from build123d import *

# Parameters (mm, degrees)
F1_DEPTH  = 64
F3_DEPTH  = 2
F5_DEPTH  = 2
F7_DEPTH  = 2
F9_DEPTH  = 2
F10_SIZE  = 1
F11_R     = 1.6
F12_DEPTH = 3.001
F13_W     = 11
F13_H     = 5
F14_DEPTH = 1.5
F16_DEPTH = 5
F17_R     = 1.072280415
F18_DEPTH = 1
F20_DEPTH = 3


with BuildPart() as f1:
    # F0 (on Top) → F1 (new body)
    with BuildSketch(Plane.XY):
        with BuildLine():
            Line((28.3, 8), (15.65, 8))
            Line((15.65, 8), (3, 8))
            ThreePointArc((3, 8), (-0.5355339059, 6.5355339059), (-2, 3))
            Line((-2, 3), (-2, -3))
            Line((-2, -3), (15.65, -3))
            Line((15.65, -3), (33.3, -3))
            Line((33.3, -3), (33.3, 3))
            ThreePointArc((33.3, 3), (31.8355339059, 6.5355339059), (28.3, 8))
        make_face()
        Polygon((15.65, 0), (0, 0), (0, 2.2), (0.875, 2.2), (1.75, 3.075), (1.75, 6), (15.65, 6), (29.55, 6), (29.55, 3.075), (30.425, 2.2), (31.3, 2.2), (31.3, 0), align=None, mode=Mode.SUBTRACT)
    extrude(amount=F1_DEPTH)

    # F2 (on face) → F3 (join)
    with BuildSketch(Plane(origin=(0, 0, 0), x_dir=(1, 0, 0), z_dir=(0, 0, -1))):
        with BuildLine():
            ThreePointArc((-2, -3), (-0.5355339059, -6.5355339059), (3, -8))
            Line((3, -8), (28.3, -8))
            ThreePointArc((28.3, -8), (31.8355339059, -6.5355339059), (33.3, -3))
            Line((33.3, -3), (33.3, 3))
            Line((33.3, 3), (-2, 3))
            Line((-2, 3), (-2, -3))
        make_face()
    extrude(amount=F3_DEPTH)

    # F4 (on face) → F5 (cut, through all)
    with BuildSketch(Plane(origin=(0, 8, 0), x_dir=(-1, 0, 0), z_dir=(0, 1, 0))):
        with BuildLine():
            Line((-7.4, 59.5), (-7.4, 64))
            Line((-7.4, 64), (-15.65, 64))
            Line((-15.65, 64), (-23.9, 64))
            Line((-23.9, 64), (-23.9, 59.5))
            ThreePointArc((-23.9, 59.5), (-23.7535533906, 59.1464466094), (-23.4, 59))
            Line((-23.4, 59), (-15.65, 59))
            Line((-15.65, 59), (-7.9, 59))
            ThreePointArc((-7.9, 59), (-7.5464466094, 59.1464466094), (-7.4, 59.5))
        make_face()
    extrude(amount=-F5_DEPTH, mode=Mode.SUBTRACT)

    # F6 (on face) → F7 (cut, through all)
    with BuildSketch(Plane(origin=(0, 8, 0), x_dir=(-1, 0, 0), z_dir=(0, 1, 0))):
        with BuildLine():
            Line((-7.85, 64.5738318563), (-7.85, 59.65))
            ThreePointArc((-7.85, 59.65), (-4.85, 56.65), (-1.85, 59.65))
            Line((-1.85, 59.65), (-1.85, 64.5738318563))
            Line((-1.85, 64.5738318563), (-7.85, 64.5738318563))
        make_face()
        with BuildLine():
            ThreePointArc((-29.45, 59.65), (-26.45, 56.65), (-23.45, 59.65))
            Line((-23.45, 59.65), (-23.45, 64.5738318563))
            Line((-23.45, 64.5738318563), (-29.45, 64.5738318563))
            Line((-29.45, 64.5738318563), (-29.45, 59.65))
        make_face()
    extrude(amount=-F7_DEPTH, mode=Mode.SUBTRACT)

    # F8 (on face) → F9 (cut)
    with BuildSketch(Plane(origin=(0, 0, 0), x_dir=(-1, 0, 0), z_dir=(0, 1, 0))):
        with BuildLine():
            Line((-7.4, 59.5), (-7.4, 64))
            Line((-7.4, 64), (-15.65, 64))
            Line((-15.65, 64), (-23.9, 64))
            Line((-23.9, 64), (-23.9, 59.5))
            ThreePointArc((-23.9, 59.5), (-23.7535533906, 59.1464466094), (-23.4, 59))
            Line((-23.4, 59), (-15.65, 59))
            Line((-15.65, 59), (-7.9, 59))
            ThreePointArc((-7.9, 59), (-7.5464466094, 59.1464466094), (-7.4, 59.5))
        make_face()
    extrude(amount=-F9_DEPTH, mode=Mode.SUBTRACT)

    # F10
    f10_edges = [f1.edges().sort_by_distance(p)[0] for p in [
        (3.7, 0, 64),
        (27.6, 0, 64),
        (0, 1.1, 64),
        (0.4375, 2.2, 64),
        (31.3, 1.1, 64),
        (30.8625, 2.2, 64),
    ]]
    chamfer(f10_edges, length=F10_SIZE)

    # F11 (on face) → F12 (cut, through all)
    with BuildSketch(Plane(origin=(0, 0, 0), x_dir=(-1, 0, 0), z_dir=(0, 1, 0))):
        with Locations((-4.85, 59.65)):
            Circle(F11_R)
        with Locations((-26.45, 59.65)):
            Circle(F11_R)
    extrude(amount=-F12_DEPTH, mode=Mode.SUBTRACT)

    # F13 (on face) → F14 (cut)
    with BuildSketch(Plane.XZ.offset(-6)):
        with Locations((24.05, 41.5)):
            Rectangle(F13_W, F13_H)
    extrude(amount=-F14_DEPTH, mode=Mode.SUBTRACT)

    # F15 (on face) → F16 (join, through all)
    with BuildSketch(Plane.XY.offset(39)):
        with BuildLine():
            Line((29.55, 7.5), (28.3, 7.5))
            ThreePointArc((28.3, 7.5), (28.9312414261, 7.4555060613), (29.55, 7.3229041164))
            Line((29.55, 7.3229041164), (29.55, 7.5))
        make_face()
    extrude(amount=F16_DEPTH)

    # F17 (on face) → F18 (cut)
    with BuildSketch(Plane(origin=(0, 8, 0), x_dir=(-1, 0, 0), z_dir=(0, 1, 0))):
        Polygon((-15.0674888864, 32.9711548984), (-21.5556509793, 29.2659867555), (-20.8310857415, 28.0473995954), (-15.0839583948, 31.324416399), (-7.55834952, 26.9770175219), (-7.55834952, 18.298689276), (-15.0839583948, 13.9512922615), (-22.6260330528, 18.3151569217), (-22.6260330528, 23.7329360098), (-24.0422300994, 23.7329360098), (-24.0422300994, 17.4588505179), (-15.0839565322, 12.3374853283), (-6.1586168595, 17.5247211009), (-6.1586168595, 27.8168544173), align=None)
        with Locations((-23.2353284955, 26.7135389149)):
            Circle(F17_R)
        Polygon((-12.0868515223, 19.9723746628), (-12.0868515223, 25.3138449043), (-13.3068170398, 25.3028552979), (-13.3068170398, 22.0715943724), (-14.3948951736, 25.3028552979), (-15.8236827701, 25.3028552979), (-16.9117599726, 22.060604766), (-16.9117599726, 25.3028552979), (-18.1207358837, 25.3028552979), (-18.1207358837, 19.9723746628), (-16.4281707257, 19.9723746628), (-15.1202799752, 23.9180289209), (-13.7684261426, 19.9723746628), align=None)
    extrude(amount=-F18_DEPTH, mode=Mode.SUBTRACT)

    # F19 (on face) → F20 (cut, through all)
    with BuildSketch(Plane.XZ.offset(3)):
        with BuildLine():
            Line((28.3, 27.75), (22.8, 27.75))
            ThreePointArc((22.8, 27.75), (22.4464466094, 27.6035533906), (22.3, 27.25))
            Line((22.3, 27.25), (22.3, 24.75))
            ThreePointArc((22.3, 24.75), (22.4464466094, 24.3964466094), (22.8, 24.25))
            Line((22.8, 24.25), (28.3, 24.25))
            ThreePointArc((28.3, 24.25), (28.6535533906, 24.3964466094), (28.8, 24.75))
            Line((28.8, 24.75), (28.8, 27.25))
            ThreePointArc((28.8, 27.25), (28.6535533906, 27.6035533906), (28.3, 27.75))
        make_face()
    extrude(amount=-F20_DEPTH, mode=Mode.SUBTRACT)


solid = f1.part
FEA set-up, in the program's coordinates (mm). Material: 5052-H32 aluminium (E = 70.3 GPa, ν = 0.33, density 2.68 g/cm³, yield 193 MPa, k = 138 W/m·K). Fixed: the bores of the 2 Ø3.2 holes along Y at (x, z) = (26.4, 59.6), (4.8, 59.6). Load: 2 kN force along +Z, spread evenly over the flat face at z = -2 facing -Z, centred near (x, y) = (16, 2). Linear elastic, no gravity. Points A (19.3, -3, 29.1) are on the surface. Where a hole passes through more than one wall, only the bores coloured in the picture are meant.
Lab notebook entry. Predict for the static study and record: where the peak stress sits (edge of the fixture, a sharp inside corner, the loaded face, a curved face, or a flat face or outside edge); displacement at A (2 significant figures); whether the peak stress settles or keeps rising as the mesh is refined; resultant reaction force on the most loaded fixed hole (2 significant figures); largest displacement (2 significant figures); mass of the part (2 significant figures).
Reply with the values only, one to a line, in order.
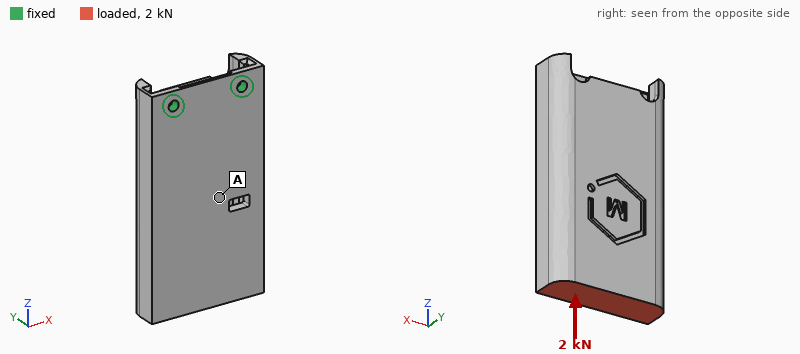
edge of the fixture
0.19 mm
keeps rising
1.0 kN
0.43 mm
35 g
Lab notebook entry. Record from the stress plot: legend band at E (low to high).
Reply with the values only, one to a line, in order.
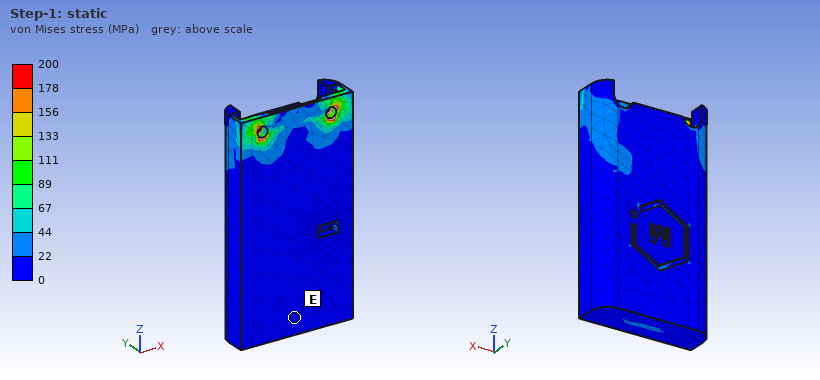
0 to 22 MPa
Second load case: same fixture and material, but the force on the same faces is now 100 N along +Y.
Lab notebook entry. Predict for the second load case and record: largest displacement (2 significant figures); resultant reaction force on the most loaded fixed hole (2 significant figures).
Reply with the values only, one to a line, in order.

0.36 mm
77 N
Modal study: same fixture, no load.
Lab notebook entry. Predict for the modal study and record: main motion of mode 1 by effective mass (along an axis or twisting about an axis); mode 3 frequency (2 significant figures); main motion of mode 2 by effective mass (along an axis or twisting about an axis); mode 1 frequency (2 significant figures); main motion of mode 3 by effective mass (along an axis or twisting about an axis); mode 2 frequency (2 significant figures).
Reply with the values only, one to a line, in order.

along Y
4200 Hz
along X
790 Hz
along X
3900 Hz
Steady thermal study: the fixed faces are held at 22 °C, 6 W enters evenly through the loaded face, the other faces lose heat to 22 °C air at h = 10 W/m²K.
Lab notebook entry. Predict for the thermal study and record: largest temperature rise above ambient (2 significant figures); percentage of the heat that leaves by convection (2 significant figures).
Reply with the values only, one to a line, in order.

15 K
14 %
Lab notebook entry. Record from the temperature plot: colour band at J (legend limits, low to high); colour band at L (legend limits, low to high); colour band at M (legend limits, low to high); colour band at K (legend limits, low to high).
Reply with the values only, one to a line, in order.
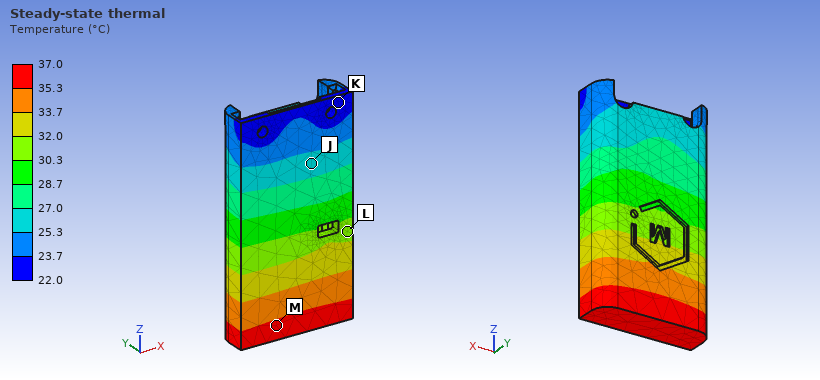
25.3 to 27.0 °C
30.3 to 32.0 °C
35.3 to 37.0 °C
22.0 to 23.7 °C
